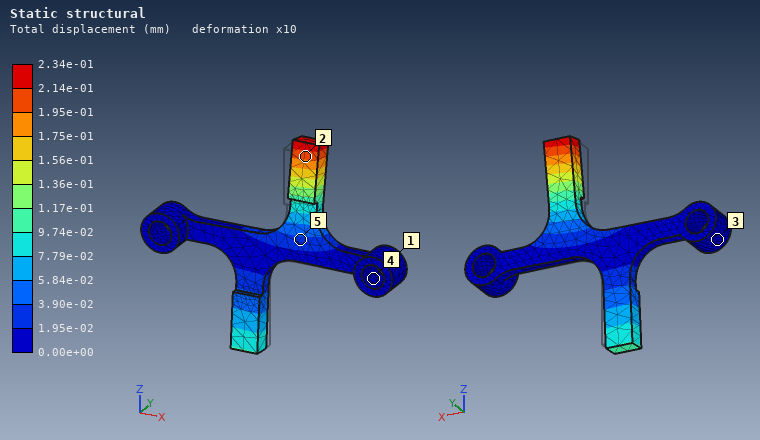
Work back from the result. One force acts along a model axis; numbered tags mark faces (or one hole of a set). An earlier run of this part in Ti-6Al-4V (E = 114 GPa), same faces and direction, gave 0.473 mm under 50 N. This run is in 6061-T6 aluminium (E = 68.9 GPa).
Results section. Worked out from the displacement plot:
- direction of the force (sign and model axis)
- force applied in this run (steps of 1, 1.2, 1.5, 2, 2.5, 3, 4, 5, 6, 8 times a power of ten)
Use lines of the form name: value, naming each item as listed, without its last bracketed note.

direction of the force: +Y
force applied in this run: 15 N
